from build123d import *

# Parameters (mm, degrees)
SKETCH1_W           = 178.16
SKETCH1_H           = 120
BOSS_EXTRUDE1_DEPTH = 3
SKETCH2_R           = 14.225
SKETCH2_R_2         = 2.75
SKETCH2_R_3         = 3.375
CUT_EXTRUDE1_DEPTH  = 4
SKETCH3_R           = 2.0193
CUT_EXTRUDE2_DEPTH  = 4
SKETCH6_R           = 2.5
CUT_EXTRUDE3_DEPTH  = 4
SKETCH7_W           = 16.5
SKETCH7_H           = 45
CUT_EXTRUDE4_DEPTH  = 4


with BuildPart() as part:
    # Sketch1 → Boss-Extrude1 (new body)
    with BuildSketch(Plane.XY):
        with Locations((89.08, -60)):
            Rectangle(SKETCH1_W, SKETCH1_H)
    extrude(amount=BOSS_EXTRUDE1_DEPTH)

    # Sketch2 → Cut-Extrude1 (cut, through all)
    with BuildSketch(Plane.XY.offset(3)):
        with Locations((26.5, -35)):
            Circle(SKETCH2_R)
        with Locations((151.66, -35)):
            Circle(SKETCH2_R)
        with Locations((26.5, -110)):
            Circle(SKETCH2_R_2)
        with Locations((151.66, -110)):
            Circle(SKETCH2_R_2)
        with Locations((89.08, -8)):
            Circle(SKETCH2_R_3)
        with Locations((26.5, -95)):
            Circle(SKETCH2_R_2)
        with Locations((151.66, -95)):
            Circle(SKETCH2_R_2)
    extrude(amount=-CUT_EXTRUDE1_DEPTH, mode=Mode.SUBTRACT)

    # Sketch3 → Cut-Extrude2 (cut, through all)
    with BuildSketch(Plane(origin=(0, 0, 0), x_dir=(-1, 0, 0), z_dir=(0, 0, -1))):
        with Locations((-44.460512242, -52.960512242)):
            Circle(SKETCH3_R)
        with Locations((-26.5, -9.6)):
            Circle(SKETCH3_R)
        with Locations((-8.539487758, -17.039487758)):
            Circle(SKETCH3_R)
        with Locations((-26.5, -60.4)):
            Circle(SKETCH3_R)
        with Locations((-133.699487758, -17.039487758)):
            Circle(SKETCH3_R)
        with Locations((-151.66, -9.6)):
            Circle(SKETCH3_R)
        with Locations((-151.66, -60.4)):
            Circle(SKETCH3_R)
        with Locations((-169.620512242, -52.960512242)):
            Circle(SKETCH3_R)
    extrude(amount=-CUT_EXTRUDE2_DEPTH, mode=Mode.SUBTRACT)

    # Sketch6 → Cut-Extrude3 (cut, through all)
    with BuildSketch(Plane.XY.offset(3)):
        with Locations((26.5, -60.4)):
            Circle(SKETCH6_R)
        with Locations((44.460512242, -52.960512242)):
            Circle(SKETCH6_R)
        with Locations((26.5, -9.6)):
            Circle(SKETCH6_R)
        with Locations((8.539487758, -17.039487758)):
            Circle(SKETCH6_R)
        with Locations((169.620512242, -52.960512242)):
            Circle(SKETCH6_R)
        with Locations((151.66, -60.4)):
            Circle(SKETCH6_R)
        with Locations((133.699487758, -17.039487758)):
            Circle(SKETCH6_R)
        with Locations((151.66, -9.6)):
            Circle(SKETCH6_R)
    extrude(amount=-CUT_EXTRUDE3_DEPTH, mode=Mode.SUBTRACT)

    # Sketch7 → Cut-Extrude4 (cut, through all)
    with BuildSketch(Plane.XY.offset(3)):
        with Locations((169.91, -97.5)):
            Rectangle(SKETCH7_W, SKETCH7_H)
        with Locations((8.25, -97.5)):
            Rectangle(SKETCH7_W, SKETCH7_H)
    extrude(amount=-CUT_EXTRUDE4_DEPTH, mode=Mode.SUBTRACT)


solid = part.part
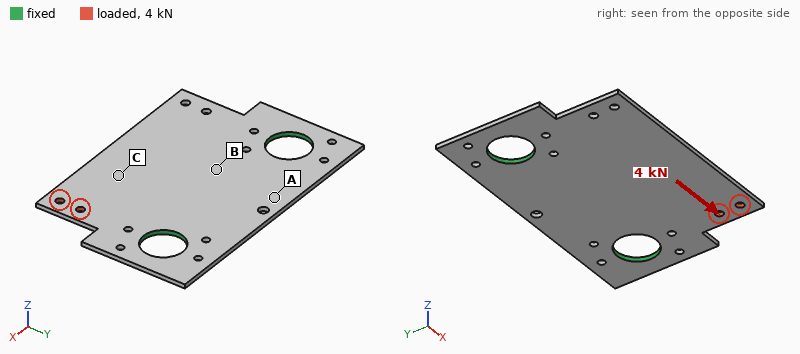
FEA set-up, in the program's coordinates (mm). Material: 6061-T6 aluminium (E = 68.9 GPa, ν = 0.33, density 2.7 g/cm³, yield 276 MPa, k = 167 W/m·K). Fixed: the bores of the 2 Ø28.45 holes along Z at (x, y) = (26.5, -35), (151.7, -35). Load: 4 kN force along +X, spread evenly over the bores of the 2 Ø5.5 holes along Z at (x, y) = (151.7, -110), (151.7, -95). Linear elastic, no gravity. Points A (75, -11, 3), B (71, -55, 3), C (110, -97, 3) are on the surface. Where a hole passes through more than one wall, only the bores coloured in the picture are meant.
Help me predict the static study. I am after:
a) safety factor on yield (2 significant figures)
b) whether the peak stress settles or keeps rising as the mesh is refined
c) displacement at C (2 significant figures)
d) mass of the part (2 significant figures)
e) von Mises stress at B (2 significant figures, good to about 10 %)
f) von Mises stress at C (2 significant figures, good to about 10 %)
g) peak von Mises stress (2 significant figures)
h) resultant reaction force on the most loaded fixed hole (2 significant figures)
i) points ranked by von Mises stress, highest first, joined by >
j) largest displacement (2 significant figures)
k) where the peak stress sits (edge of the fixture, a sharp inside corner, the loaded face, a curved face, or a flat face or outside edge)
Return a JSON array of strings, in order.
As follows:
["3.0", "settles", "26 µm", "150 g", "14 MPa", "23 MPa", "94 MPa", "2.8 kN", "C > B > A", "55 µm", "the loaded face"]
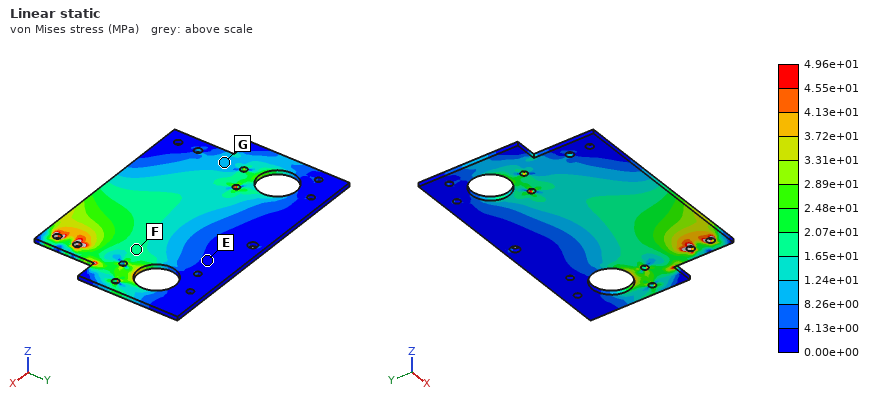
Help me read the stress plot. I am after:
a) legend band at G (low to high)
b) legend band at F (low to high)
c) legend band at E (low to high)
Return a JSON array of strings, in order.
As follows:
["8.26e+00 to 1.24e+01 MPa", "1.65e+01 to 2.07e+01 MPa", "0.00e+00 to 4.13e+00 MPa"]
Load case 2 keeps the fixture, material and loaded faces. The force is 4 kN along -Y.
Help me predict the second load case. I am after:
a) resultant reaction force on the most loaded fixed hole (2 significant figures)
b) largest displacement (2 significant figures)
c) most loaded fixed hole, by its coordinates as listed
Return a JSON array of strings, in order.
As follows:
["4.0 kN", "48 µm", "(151.7, -35)"]
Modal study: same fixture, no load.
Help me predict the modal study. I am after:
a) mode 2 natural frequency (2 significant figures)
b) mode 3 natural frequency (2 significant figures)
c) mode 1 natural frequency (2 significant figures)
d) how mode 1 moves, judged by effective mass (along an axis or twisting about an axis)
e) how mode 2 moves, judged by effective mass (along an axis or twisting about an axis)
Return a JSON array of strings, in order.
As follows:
["770 Hz", "1300 Hz", "410 Hz", "along Z", "twisting about Y"]
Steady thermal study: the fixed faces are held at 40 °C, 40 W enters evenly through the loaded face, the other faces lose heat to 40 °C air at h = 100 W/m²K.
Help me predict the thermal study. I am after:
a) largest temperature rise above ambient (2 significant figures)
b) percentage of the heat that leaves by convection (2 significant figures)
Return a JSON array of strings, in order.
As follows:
["61 K", "63 %"]
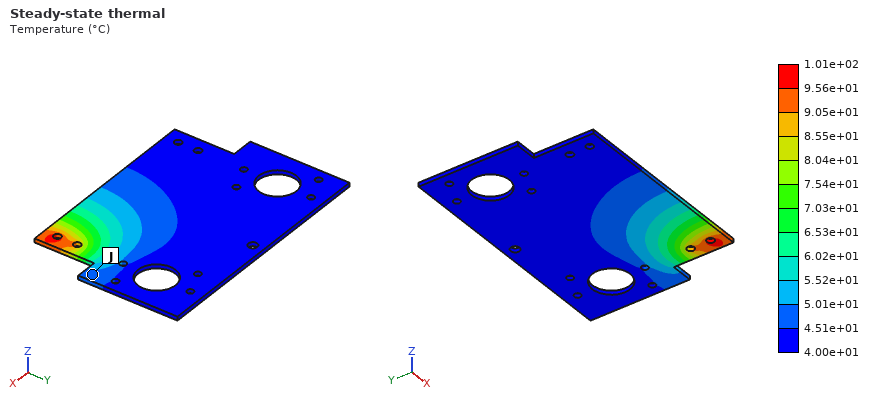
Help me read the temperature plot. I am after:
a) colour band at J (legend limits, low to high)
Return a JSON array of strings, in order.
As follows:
["4.51e+01 to 5.01e+01 °C"]
